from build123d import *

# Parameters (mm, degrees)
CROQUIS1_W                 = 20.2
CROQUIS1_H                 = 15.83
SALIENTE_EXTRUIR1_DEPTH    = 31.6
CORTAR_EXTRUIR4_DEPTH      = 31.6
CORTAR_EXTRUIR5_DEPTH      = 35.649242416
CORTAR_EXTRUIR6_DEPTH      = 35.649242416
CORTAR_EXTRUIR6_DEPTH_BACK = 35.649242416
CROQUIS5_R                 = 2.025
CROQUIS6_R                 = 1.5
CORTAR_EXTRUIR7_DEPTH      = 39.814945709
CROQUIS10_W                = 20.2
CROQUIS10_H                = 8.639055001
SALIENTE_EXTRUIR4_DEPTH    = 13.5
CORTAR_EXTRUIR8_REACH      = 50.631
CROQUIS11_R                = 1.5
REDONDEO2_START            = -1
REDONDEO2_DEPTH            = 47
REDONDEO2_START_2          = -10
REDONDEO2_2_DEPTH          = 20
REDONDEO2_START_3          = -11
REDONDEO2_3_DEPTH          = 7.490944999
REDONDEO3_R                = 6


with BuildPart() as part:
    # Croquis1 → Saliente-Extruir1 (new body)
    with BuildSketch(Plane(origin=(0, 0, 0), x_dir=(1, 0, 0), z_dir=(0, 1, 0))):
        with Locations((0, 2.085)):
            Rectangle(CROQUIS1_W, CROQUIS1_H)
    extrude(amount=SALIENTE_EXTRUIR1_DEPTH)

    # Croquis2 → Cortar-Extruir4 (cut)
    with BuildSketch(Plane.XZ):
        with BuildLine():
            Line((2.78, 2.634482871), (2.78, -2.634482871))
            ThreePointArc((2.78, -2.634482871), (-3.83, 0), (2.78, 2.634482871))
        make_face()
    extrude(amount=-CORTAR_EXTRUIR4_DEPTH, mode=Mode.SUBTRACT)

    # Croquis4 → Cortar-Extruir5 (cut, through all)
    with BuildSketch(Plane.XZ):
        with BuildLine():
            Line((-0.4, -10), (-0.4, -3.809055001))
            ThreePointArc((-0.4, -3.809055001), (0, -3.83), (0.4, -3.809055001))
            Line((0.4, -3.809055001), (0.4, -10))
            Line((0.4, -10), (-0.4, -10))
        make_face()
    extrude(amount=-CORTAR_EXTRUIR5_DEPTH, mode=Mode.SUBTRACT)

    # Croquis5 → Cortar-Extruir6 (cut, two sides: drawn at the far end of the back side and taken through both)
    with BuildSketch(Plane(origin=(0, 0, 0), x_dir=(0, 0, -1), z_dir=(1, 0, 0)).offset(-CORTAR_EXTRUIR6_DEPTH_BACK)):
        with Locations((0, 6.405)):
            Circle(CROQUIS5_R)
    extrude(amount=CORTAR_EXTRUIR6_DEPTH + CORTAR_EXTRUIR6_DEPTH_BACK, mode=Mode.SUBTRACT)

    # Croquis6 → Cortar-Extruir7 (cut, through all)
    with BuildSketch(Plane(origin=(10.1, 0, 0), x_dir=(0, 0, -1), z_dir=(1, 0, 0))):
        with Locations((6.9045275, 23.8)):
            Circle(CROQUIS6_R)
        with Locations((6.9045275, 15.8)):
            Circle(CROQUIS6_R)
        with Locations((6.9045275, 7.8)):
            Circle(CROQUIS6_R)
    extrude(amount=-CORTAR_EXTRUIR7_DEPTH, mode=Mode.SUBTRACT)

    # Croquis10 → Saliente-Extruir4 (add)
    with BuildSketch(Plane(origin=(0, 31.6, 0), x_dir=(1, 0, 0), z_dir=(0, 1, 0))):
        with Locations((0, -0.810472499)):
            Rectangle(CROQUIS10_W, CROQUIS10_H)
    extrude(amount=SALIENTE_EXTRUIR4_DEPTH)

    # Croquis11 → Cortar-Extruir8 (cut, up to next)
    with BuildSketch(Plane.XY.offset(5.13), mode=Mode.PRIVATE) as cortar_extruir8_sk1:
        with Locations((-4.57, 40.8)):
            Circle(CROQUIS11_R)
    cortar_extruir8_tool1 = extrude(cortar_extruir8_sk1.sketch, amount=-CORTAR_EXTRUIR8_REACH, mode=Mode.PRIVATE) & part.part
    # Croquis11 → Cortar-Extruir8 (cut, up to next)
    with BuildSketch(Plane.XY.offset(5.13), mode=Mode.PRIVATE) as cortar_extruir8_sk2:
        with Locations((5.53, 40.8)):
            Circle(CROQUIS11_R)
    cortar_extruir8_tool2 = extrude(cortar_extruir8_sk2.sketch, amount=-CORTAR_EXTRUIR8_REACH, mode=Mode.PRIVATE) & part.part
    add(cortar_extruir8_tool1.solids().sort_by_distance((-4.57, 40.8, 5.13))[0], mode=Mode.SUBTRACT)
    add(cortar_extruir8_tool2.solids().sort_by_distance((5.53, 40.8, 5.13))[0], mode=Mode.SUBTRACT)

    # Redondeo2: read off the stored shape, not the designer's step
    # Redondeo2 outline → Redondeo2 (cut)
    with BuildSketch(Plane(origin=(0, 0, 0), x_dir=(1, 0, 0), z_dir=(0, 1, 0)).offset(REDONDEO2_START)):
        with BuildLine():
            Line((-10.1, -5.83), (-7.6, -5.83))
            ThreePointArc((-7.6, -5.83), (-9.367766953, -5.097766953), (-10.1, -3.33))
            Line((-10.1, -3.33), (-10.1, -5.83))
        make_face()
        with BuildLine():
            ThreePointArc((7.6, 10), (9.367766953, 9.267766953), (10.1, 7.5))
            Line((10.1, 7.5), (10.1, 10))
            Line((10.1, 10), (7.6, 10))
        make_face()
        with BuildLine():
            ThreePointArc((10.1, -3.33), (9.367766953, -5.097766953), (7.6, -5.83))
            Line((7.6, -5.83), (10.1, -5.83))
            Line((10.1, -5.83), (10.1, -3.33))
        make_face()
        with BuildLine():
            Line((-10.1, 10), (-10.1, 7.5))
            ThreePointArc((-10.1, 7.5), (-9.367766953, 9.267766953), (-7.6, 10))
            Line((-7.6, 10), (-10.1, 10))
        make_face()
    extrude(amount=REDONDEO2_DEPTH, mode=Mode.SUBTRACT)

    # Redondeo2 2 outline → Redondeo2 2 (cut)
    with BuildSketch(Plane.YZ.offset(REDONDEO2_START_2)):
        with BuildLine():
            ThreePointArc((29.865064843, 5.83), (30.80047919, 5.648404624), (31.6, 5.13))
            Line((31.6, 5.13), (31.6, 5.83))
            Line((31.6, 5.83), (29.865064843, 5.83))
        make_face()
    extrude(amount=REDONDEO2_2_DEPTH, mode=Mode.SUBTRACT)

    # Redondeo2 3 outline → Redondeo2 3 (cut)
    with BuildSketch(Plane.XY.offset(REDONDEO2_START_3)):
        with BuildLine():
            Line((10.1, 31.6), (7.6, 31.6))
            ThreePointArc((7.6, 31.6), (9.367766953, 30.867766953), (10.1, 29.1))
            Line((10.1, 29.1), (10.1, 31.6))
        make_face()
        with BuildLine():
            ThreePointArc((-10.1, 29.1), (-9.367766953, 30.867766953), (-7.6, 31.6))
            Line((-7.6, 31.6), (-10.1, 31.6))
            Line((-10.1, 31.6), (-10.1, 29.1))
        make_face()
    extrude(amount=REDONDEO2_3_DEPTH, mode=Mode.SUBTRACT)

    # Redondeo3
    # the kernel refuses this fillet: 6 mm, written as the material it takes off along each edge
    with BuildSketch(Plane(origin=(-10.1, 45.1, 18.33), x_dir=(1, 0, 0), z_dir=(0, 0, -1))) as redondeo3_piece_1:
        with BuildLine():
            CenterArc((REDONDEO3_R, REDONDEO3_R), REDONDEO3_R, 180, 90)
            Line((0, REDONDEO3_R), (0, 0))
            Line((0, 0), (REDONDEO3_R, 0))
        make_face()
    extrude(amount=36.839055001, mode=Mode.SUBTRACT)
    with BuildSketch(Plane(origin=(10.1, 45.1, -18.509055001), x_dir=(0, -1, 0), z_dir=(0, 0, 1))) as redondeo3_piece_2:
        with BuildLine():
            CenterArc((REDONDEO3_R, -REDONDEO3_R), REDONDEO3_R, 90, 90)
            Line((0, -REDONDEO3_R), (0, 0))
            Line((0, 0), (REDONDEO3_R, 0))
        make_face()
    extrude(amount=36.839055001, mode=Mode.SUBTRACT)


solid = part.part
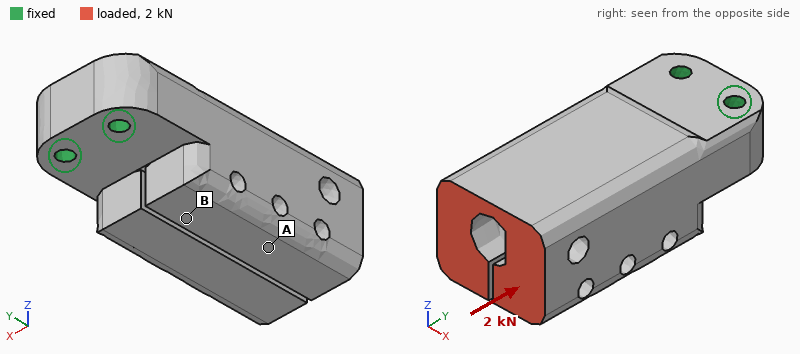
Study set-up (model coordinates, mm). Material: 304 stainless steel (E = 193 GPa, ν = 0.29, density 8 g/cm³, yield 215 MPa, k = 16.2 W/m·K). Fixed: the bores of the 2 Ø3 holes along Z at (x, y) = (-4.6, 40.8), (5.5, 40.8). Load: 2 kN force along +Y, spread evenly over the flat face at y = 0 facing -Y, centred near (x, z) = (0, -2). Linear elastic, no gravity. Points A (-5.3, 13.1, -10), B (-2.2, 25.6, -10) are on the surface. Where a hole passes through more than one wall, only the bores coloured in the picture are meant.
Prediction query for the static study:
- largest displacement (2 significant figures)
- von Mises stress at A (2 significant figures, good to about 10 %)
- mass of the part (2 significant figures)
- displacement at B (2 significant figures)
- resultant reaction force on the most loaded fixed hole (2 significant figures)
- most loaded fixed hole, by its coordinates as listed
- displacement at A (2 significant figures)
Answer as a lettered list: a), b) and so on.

a) 17 µm
b) 13 MPa
c) 79 g
d) 7.4 µm
e) 1.1 kN
f) (-4.6, 40.8)
g) 12 µm
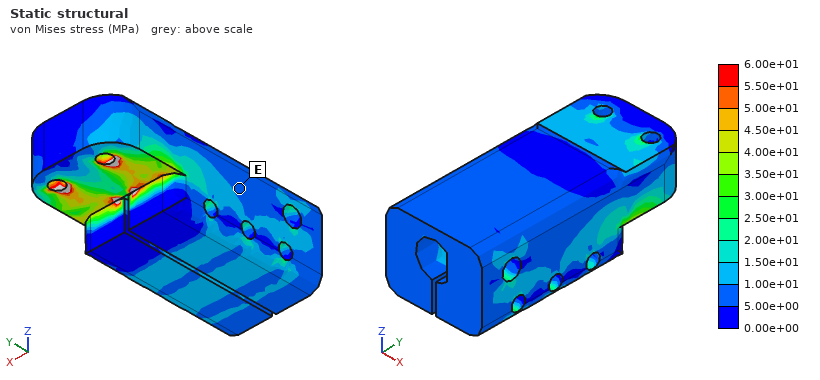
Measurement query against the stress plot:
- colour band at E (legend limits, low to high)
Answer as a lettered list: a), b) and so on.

a) 5.00e+00 to 1.00e+01 MPa
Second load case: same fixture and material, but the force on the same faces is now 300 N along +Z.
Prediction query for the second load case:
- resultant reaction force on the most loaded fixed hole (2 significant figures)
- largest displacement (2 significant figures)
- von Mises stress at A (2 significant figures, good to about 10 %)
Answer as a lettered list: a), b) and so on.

a) 160 N
b) 29 µm
c) 7.5 MPa
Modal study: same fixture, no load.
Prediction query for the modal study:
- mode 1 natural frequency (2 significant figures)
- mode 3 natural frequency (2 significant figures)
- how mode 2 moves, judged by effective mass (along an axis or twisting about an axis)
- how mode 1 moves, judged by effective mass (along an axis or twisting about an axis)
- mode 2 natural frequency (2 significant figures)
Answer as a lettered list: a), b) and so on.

a) 3400 Hz
b) 9100 Hz
c) along X
d) along Z
e) 5000 Hz
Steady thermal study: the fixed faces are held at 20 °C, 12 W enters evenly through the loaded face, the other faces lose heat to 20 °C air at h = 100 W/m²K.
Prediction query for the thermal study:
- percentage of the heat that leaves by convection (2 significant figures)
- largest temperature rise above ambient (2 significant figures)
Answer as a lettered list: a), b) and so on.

a) 84 %
b) 58 K
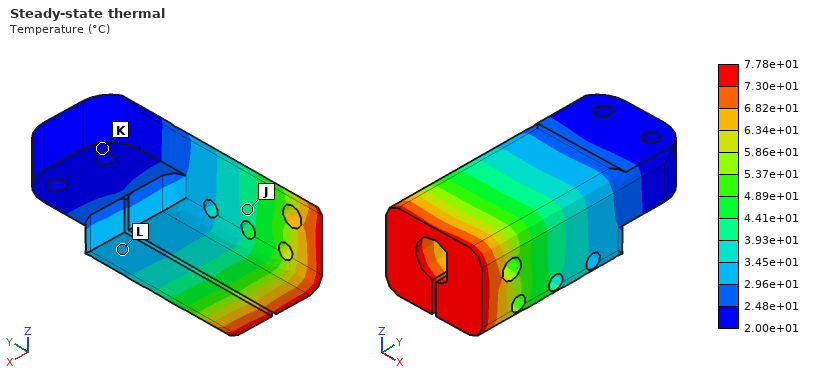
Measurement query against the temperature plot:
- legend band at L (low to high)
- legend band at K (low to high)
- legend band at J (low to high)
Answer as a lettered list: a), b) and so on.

a) 2.96e+01 to 3.45e+01 °C
b) 2.00e+01 to 2.48e+01 °C
c) 3.93e+01 to 4.41e+01 °C
